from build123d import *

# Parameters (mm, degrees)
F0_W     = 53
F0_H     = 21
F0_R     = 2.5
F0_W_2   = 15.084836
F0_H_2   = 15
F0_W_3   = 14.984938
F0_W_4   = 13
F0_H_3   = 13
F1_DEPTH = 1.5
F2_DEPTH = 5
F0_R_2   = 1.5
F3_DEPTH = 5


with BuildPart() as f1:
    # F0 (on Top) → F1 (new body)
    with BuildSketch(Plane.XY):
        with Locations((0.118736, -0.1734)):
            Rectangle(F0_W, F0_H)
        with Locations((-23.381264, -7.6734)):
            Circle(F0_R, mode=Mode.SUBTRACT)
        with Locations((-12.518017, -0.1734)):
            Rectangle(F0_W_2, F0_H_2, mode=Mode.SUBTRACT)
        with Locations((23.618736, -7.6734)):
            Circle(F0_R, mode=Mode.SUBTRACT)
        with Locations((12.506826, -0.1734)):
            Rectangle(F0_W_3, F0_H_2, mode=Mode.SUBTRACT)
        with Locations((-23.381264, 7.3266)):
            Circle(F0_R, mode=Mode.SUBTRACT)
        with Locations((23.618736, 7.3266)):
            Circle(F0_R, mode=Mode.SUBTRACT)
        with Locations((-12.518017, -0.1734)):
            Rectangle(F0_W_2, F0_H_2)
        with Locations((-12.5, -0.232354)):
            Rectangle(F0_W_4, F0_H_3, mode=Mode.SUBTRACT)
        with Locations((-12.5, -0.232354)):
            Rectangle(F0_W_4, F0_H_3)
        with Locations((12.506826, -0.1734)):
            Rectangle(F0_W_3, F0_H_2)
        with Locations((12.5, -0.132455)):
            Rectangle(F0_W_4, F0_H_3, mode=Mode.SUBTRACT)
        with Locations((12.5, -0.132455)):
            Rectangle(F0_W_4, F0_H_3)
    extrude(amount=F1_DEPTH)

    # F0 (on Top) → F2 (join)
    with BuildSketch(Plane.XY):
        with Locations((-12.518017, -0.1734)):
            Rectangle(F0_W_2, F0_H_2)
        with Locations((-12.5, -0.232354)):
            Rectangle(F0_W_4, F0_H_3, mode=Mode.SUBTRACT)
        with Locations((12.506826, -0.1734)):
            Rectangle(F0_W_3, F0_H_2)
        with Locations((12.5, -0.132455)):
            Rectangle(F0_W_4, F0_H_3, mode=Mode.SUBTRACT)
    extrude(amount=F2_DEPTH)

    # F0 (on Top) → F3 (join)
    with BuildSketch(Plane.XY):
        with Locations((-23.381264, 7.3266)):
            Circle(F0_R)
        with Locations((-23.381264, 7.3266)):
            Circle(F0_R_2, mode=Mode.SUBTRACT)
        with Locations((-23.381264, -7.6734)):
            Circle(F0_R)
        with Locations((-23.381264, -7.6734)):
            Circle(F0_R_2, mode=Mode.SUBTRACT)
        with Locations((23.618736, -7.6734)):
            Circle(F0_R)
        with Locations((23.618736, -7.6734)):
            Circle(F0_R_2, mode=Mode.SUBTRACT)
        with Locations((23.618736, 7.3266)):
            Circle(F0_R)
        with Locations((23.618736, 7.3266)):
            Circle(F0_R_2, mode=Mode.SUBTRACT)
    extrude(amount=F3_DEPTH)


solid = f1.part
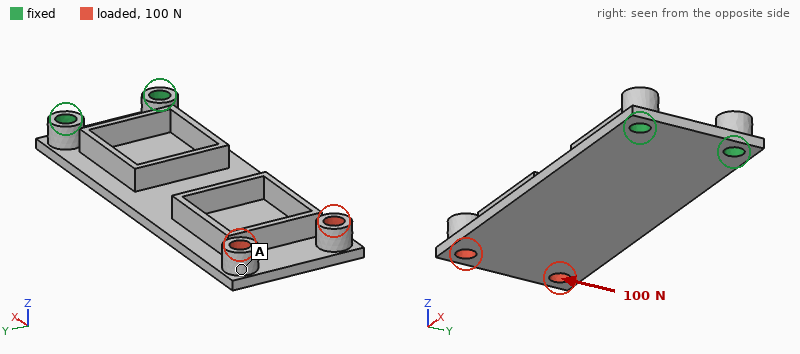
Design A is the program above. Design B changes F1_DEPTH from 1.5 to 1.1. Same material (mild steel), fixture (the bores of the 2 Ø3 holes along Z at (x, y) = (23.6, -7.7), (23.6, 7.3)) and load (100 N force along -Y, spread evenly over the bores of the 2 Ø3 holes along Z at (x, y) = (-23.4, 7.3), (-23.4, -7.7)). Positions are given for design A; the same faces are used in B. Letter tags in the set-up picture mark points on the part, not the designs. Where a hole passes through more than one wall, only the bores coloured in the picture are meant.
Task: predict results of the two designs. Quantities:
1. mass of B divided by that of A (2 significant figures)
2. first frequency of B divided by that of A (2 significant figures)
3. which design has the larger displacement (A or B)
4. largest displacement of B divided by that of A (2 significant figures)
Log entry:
0.83
0.75
B
2.0
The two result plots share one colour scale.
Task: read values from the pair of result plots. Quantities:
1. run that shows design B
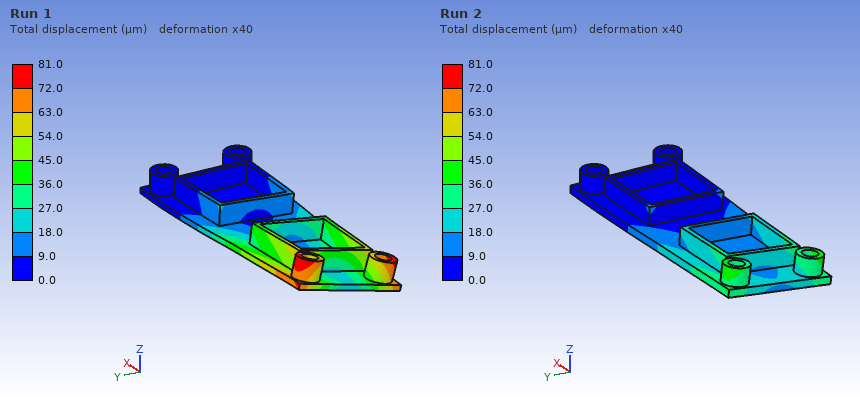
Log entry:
Run 1
